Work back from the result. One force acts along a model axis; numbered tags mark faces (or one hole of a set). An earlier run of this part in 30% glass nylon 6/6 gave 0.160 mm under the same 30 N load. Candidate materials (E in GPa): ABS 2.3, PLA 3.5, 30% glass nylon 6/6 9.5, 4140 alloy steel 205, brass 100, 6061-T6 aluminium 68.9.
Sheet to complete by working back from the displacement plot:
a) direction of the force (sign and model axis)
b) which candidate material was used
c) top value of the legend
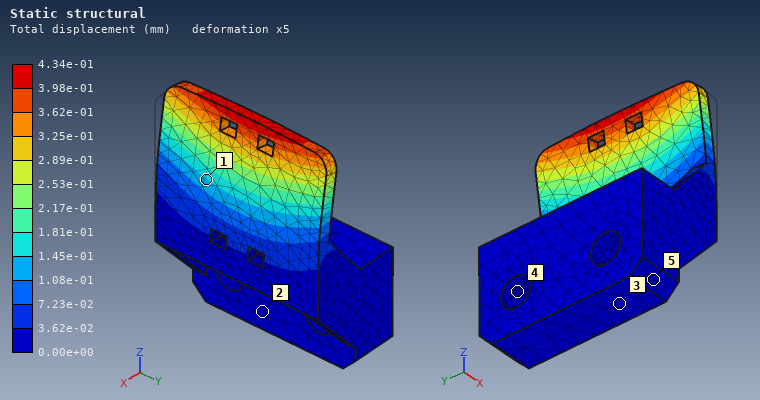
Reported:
-X
PLA
4.34e-01 mm
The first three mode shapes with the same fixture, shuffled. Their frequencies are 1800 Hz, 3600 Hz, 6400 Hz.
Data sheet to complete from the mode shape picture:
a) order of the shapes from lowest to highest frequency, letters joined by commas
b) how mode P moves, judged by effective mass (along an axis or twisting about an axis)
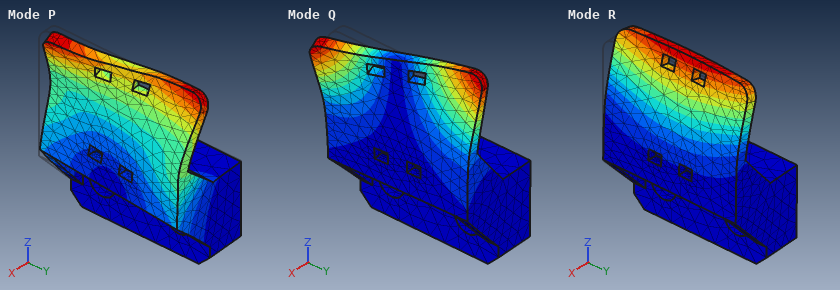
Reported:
R, Q, P
along Y
